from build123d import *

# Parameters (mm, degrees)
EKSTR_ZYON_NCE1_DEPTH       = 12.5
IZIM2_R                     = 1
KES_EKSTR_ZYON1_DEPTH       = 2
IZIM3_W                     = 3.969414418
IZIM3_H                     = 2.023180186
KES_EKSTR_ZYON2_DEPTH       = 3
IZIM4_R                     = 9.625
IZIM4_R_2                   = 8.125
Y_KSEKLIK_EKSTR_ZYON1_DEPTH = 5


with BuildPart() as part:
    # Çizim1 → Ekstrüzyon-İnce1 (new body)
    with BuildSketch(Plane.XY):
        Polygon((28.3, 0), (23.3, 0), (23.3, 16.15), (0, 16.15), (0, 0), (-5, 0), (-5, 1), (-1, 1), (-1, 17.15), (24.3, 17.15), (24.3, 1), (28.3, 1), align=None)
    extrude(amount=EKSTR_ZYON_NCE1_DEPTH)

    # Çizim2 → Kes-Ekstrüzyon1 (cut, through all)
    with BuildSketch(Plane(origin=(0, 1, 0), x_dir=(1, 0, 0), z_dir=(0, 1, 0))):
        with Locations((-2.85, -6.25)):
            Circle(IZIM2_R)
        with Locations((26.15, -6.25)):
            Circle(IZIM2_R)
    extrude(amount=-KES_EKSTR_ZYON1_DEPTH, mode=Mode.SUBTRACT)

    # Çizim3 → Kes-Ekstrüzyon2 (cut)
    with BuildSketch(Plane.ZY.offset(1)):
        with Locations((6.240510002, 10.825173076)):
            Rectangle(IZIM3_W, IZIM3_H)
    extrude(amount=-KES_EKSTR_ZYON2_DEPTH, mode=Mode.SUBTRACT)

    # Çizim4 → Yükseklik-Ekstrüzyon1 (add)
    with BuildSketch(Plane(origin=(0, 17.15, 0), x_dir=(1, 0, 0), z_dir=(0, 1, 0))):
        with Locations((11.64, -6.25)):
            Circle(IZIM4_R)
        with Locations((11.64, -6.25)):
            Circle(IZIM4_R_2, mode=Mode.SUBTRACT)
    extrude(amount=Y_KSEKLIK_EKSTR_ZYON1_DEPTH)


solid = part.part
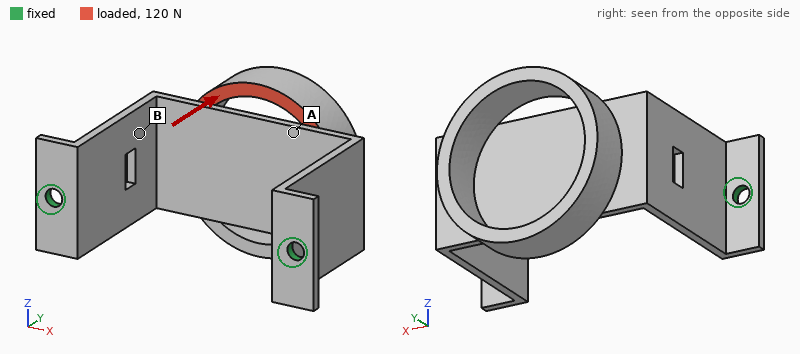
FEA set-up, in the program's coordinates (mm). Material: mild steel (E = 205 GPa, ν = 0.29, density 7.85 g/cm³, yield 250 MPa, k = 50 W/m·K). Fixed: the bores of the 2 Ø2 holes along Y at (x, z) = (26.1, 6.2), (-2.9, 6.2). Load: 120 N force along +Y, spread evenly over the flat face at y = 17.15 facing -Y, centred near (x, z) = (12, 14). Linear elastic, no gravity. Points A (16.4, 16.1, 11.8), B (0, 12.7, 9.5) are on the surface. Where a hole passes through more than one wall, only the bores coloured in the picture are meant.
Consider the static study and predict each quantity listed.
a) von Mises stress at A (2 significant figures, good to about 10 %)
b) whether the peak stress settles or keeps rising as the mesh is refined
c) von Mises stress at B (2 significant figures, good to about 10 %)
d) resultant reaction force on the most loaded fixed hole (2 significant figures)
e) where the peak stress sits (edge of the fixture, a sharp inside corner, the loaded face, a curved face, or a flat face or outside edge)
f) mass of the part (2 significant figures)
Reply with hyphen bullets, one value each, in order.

- 30 MPa
- keeps rising
- 67 MPa
- 61 N
- edge of the fixture
- 9.6 g
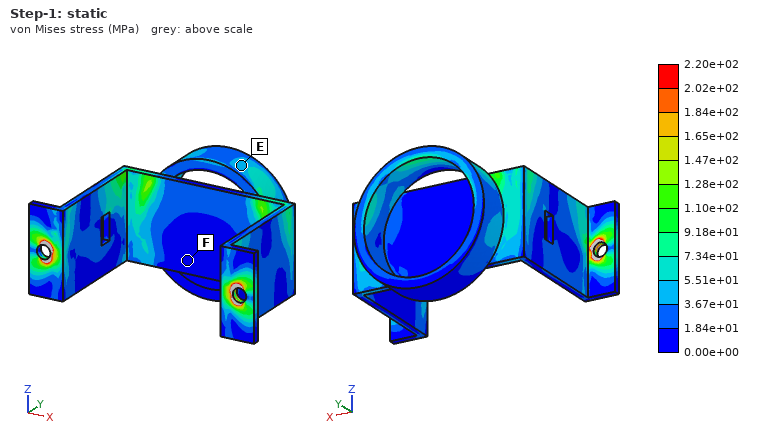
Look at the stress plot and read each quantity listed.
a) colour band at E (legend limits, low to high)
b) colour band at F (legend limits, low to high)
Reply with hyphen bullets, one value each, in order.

- 3.67e+01 to 5.51e+01 MPa
- 0.00e+00 to 1.84e+01 MPa
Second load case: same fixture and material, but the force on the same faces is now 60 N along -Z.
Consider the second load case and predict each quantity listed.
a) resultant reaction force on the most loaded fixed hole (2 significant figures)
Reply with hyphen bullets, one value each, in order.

- 30 N
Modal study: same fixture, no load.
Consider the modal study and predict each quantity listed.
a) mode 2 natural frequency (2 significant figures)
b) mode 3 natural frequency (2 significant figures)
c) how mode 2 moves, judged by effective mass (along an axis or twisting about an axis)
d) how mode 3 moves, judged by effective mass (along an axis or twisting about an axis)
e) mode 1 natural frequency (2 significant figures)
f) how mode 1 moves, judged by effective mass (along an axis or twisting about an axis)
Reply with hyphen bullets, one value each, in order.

- 1900 Hz
- 4100 Hz
- along Z
- twisting about Y
- 1600 Hz
- along X
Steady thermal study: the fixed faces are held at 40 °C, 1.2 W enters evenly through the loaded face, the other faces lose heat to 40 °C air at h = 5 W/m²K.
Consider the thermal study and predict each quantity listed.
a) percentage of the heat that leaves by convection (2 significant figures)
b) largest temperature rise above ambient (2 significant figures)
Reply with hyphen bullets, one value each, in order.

- 15 %
- 32 K
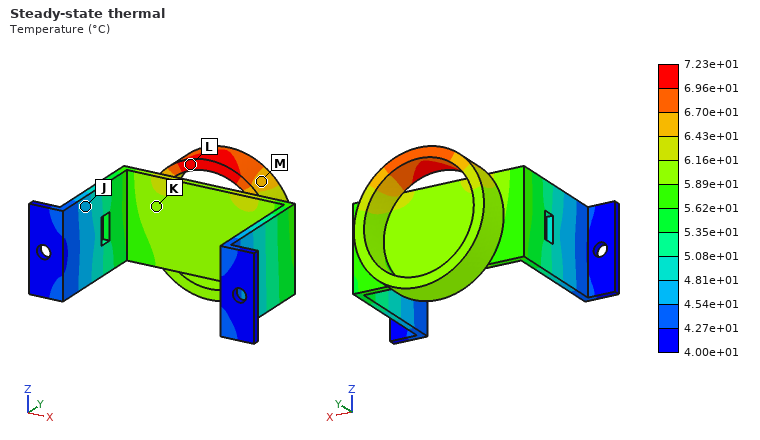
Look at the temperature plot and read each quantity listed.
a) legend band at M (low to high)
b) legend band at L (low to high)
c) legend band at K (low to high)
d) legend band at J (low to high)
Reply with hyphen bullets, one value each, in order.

- 6.43e+01 to 6.70e+01 °C
- 6.96e+01 to 7.23e+01 °C
- 5.89e+01 to 6.16e+01 °C
- 4.54e+01 to 4.81e+01 °C
